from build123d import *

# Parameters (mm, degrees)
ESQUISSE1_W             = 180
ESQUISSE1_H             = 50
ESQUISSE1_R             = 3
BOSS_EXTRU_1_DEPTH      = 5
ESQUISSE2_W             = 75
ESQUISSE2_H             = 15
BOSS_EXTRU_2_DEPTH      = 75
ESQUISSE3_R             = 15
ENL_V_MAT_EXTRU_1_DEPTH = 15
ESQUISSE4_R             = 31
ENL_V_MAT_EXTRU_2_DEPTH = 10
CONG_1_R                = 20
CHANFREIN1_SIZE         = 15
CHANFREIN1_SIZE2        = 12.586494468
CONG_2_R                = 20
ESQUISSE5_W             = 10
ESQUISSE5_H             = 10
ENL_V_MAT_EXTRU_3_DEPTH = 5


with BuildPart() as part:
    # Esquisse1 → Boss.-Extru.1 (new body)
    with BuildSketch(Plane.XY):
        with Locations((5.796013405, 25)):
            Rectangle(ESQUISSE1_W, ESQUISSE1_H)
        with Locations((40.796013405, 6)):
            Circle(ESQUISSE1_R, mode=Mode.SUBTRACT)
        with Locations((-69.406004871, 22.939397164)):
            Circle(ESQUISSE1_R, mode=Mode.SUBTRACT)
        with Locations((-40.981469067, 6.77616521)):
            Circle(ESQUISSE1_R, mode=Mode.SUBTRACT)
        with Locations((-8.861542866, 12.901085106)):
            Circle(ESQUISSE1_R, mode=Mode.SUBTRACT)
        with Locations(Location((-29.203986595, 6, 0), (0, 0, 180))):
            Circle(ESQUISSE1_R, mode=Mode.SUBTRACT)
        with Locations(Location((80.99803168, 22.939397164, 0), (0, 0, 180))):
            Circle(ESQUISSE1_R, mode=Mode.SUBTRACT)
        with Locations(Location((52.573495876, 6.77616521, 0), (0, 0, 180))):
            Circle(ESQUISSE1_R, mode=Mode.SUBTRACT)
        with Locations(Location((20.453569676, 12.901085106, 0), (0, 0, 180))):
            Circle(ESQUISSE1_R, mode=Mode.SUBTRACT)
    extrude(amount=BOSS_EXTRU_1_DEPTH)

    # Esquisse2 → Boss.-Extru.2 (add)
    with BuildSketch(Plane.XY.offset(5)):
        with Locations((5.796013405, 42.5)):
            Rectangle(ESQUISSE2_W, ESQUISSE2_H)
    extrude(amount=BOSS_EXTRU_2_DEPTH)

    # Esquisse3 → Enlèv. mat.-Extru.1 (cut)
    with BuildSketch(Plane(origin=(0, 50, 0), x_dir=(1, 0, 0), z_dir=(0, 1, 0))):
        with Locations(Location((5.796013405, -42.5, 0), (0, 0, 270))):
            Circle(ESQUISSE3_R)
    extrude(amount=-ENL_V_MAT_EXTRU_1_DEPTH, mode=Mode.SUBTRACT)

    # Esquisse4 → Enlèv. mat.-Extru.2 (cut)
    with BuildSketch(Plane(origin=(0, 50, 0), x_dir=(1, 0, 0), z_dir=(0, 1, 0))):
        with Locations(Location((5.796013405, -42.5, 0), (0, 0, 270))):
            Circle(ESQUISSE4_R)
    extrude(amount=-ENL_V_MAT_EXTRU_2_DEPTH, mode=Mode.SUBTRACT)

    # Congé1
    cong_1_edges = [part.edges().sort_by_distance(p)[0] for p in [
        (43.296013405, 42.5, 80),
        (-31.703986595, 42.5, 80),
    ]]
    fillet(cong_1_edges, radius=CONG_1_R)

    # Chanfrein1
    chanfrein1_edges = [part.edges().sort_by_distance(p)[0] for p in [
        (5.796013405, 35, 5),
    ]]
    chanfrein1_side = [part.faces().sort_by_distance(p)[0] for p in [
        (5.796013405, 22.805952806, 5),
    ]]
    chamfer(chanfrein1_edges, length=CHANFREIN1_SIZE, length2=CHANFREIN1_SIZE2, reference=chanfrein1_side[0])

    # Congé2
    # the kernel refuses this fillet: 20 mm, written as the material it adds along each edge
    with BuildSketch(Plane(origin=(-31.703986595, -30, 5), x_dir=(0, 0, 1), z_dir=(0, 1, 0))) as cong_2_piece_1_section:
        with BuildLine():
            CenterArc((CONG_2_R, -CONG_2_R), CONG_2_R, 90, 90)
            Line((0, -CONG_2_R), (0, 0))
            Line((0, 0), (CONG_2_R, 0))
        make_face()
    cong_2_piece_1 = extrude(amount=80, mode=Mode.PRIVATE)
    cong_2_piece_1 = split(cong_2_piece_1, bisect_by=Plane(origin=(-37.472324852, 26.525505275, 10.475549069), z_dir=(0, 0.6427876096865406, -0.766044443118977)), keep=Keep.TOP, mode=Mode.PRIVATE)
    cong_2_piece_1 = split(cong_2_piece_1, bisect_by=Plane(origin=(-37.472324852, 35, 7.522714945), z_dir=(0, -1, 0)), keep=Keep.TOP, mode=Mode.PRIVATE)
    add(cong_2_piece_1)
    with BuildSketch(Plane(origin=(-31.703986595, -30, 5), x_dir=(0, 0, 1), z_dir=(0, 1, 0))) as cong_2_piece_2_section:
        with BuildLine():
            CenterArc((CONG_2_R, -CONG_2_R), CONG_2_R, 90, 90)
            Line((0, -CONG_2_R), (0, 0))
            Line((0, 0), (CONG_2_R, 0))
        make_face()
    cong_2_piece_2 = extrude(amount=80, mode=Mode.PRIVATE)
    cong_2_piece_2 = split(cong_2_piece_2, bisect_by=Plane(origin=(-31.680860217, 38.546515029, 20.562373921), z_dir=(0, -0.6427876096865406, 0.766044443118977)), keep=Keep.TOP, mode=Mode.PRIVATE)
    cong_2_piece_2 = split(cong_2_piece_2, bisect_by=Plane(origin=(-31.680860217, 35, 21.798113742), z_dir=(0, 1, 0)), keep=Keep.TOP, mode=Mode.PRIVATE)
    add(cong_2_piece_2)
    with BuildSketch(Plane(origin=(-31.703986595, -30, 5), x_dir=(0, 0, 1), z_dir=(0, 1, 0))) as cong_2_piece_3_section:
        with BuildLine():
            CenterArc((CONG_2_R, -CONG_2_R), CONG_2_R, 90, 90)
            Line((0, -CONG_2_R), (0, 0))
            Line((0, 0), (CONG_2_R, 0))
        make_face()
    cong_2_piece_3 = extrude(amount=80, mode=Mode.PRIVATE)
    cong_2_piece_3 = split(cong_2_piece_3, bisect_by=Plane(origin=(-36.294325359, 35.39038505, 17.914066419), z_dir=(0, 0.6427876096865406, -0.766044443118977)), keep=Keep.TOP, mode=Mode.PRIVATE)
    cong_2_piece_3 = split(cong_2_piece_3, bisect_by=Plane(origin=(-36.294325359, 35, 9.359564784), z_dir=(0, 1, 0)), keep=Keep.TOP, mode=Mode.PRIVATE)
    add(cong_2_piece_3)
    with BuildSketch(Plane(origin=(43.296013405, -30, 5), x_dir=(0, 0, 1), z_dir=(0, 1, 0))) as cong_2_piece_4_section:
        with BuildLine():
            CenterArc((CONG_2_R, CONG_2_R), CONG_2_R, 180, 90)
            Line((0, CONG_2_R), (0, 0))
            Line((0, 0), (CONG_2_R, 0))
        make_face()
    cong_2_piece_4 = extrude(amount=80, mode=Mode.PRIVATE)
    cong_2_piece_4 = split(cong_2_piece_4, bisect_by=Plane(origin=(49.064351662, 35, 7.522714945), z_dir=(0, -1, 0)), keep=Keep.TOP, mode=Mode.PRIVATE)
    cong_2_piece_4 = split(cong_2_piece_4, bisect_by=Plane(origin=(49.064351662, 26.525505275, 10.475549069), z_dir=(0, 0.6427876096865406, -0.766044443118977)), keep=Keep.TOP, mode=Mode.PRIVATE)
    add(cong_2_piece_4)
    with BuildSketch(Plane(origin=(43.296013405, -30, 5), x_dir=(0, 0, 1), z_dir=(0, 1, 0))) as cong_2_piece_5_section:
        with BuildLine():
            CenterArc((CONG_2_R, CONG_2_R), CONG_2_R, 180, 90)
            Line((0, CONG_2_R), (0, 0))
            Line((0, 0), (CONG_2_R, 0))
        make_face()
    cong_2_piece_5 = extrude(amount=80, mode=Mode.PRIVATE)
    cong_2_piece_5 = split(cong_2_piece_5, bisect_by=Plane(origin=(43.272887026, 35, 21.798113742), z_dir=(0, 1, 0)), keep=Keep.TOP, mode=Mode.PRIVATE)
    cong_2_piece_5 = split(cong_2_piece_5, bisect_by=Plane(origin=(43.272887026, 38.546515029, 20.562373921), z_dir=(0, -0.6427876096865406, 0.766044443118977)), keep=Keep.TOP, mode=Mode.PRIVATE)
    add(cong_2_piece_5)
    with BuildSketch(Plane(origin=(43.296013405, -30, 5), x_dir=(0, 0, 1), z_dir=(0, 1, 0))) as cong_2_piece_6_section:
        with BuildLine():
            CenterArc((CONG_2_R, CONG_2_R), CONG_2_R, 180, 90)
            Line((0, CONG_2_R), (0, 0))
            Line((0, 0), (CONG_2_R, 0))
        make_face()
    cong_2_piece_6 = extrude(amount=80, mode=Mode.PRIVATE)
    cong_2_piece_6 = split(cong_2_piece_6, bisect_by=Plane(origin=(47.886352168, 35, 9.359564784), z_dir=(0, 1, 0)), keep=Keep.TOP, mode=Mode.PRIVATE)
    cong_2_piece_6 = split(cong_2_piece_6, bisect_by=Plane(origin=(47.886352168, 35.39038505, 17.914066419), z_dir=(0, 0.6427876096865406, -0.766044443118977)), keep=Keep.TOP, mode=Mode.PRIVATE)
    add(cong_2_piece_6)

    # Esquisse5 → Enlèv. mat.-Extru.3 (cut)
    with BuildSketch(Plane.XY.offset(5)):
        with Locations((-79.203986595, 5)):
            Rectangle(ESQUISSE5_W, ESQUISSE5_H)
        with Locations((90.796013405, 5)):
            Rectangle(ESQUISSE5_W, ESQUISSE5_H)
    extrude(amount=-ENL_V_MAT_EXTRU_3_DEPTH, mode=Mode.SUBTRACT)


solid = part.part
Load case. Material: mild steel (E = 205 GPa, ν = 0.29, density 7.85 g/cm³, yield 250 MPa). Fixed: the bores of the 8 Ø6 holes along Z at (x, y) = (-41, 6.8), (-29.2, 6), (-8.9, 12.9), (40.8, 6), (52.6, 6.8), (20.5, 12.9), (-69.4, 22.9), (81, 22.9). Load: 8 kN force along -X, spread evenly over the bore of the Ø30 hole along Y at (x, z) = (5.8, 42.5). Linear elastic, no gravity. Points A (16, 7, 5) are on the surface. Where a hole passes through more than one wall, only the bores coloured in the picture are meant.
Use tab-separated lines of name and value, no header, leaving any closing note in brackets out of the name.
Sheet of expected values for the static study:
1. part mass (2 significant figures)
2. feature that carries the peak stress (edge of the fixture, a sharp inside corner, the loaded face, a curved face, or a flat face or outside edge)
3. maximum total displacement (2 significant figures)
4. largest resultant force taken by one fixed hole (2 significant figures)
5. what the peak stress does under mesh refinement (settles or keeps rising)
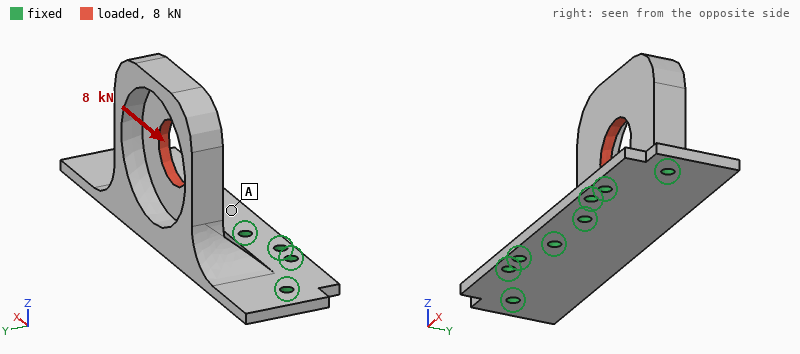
part mass	800 g
feature that carries the peak stress	edge of the fixture
maximum total displacement	92 µm
largest resultant force taken by one fixed hole	2.1 kN
what the peak stress does under mesh refinement	keeps rising
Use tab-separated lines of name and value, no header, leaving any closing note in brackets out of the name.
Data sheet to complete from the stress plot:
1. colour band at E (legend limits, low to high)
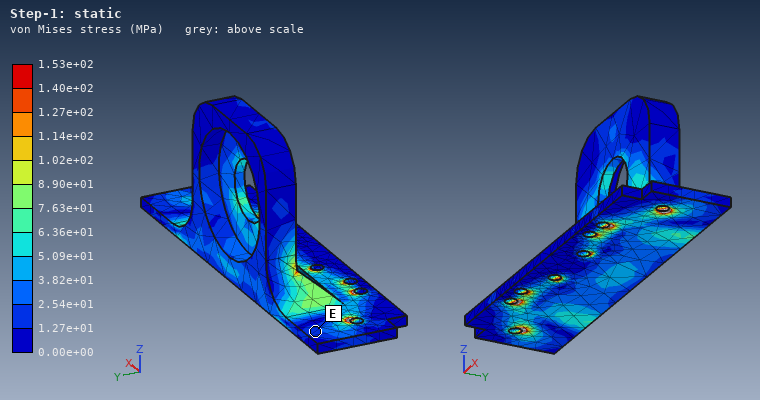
colour band at E	1.27e+01 to 2.54e+01 MPa
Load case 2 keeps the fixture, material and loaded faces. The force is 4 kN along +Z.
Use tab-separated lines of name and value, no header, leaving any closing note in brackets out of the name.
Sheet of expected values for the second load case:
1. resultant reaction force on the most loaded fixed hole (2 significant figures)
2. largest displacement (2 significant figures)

resultant reaction force on the most loaded fixed hole	1.4 kN
largest displacement	0.19 mm
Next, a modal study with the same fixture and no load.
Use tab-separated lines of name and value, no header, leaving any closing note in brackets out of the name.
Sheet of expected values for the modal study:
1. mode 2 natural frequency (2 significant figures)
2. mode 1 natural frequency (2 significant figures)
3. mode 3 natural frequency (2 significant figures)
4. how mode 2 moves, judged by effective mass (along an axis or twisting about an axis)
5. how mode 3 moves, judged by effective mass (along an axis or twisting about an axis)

mode 2 natural frequency	2500 Hz
mode 1 natural frequency	830 Hz
mode 3 natural frequency	3300 Hz
how mode 2 moves, judged by effective mass	along X
how mode 3 moves, judged by effective mass	along Z
